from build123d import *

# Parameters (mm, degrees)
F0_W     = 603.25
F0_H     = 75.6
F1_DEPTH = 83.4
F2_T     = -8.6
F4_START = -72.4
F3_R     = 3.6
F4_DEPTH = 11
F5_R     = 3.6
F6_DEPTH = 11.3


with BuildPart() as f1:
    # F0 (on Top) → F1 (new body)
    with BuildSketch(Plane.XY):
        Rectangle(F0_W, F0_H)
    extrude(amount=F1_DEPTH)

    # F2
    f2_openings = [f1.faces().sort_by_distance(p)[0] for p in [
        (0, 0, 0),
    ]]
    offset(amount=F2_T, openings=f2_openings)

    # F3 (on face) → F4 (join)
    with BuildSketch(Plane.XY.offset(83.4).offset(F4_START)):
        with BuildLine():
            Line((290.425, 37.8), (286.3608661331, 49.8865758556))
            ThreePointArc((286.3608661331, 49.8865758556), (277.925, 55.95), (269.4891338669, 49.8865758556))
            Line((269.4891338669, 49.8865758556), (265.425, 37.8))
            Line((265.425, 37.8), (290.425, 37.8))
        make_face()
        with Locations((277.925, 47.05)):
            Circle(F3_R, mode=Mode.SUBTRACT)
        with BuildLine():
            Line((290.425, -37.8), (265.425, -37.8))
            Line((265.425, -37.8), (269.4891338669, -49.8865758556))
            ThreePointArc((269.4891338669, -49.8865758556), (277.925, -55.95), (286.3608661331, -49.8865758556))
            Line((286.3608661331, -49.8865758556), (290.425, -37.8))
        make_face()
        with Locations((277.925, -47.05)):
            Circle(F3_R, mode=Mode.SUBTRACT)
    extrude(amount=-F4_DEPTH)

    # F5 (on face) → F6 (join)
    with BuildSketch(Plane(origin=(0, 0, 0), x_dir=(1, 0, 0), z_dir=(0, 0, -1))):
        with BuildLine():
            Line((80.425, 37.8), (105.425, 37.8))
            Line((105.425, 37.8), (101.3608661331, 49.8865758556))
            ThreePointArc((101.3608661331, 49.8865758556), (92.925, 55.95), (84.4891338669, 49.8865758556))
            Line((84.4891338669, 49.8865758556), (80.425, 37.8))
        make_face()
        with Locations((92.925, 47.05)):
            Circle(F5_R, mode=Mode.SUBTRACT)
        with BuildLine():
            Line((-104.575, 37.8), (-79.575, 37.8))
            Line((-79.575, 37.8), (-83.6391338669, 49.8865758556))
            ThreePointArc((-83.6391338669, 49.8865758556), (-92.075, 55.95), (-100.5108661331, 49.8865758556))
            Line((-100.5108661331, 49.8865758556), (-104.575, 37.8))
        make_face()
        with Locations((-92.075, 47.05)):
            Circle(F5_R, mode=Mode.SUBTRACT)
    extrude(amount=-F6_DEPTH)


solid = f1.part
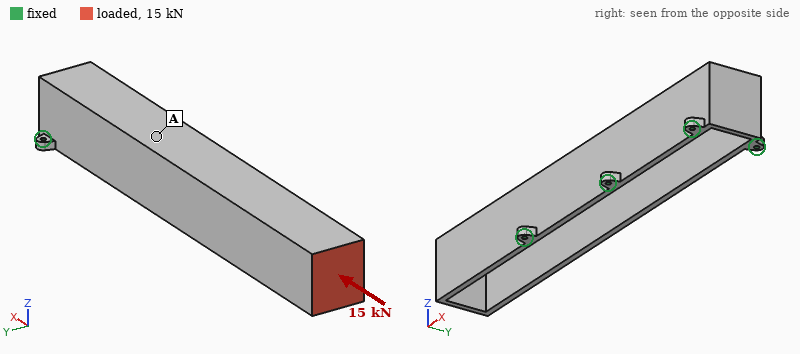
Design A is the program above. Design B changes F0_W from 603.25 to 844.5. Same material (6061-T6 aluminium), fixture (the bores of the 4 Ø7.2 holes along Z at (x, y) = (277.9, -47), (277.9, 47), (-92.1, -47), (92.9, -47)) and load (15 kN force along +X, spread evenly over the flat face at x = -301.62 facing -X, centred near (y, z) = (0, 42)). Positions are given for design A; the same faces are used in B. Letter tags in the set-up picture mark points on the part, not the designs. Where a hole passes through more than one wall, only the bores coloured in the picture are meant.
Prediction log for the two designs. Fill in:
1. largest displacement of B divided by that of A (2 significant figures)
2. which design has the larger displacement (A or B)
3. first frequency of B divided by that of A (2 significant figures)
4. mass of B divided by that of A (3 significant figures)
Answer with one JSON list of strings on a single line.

["1.4", "B", "0.64", "1.37"]
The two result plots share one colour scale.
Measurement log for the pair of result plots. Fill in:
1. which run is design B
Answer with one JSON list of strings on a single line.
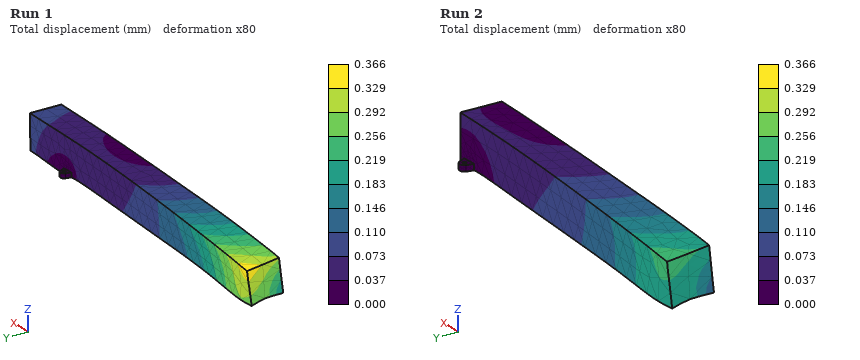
["Run 1"]
